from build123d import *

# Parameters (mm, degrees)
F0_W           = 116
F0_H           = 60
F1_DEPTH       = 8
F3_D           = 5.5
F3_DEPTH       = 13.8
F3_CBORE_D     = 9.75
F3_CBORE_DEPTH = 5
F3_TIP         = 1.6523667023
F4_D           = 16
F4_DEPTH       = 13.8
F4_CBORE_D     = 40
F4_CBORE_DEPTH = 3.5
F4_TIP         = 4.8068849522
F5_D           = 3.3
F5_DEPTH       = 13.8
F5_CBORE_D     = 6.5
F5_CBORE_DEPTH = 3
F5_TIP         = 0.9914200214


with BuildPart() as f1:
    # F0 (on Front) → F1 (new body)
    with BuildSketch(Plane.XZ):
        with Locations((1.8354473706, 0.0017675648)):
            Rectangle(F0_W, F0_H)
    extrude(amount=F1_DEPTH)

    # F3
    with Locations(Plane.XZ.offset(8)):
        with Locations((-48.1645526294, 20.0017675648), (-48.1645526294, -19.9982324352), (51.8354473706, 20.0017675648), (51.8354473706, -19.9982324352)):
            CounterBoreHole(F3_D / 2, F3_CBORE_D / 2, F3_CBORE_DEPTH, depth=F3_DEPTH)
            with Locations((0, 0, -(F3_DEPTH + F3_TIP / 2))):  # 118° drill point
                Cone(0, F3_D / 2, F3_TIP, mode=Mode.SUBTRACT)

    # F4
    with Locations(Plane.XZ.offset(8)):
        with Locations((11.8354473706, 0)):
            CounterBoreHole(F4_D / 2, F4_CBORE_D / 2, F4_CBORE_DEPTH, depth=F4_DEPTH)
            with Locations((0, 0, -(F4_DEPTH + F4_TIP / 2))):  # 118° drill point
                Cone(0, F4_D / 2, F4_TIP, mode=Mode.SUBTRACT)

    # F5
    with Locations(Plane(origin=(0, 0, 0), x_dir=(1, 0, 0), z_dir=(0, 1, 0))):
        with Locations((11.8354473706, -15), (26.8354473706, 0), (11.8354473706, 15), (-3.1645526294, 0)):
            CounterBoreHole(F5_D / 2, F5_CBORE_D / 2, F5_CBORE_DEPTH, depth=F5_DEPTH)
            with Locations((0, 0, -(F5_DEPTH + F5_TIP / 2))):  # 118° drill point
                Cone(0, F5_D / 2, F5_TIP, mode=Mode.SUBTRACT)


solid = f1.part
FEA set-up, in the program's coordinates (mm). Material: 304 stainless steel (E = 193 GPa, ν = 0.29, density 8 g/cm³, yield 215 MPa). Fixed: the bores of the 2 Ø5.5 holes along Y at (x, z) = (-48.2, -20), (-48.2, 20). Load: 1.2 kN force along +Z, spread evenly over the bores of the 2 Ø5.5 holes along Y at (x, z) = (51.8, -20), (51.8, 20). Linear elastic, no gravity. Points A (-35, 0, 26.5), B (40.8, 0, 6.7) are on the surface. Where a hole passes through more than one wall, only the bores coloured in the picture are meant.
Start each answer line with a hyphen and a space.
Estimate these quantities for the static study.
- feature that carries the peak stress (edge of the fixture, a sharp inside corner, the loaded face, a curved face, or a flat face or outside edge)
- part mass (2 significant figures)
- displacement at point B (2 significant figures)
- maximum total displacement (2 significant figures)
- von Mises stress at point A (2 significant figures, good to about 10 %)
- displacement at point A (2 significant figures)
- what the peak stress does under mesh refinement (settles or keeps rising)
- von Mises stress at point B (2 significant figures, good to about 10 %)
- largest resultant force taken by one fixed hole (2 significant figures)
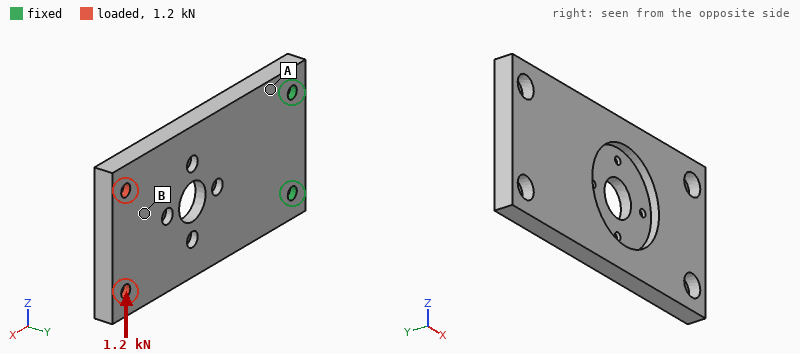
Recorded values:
- edge of the fixture
- 390 g
- 30 µm
- 43 µm
- 28 MPa
- 6.4 µm
- keeps rising
- 11 MPa
- 2.9 kN
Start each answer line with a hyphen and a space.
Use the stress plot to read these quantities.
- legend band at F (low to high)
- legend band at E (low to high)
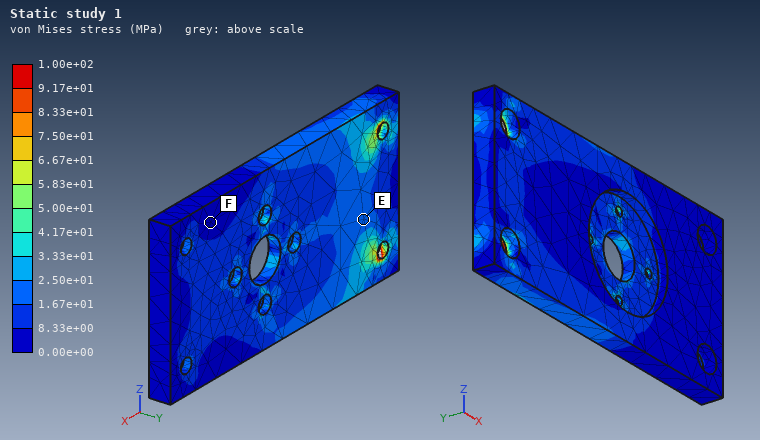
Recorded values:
- 0.00e+00 to 8.33e+00 MPa
- 1.67e+01 to 2.50e+01 MPa
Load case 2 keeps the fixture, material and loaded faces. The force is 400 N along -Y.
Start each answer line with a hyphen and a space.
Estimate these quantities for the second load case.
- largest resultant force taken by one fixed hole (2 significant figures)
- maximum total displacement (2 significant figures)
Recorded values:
- 330 N
- 0.60 mm
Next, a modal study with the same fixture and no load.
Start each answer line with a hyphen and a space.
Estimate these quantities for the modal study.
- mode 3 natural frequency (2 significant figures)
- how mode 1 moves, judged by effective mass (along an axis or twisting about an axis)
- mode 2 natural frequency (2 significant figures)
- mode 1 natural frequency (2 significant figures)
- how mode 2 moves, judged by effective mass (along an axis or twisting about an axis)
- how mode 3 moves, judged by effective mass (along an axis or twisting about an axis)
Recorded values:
- 2400 Hz
- along Y
- 1700 Hz
- 400 Hz
- twisting about X
- along Y
